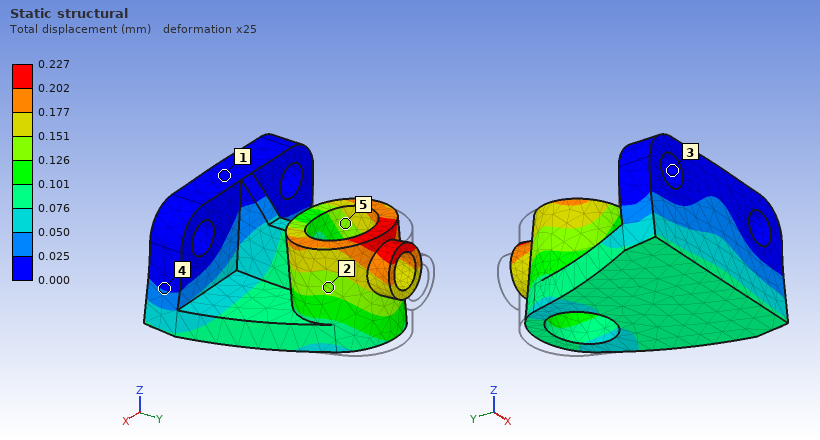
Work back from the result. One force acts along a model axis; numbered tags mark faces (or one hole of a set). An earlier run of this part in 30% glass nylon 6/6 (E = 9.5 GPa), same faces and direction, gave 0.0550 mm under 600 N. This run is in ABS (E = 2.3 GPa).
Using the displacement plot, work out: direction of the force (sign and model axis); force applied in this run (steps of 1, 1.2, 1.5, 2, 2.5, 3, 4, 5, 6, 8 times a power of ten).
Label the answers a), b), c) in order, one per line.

a) -Y
b) 600 N
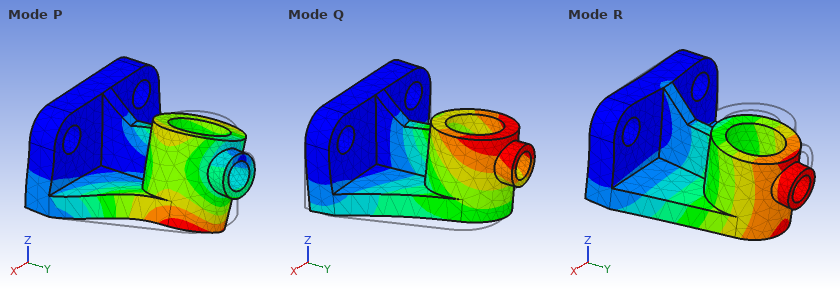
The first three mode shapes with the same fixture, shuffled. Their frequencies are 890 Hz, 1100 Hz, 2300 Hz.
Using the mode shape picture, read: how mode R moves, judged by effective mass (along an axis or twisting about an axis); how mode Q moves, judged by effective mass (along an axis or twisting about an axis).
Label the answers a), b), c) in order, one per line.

a) along Z
b) along X
